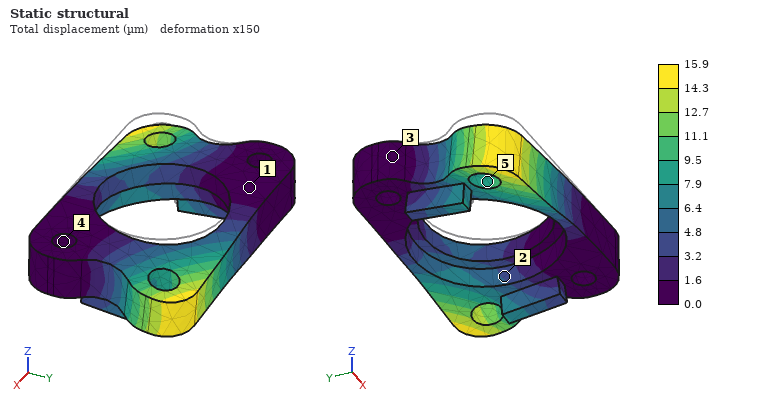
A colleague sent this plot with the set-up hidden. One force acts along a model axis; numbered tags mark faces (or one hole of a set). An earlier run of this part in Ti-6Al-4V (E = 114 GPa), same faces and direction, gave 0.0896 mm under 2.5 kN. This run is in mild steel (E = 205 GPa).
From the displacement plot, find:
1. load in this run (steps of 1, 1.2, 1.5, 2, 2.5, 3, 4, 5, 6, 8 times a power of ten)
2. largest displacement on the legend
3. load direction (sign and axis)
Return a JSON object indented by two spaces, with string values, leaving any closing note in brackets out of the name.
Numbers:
{
  "load in this run": "800 N",
  "largest displacement on the legend": "15.9 µm",
  "load direction": "-Z"
}
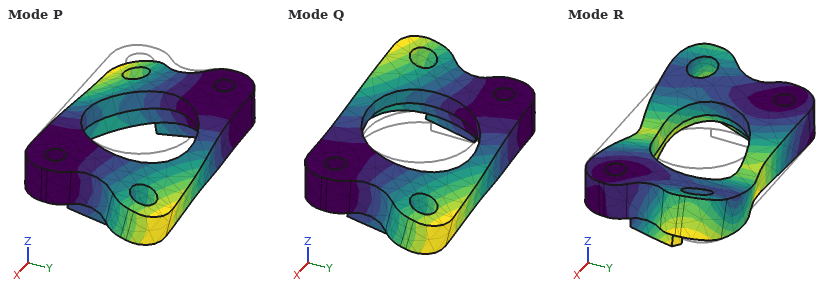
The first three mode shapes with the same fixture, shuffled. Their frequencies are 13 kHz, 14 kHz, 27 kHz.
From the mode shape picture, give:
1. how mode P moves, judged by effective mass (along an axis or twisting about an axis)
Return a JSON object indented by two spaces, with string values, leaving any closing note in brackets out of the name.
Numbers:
{
  "how mode P moves, judged by effective mass": "along Z"
}
